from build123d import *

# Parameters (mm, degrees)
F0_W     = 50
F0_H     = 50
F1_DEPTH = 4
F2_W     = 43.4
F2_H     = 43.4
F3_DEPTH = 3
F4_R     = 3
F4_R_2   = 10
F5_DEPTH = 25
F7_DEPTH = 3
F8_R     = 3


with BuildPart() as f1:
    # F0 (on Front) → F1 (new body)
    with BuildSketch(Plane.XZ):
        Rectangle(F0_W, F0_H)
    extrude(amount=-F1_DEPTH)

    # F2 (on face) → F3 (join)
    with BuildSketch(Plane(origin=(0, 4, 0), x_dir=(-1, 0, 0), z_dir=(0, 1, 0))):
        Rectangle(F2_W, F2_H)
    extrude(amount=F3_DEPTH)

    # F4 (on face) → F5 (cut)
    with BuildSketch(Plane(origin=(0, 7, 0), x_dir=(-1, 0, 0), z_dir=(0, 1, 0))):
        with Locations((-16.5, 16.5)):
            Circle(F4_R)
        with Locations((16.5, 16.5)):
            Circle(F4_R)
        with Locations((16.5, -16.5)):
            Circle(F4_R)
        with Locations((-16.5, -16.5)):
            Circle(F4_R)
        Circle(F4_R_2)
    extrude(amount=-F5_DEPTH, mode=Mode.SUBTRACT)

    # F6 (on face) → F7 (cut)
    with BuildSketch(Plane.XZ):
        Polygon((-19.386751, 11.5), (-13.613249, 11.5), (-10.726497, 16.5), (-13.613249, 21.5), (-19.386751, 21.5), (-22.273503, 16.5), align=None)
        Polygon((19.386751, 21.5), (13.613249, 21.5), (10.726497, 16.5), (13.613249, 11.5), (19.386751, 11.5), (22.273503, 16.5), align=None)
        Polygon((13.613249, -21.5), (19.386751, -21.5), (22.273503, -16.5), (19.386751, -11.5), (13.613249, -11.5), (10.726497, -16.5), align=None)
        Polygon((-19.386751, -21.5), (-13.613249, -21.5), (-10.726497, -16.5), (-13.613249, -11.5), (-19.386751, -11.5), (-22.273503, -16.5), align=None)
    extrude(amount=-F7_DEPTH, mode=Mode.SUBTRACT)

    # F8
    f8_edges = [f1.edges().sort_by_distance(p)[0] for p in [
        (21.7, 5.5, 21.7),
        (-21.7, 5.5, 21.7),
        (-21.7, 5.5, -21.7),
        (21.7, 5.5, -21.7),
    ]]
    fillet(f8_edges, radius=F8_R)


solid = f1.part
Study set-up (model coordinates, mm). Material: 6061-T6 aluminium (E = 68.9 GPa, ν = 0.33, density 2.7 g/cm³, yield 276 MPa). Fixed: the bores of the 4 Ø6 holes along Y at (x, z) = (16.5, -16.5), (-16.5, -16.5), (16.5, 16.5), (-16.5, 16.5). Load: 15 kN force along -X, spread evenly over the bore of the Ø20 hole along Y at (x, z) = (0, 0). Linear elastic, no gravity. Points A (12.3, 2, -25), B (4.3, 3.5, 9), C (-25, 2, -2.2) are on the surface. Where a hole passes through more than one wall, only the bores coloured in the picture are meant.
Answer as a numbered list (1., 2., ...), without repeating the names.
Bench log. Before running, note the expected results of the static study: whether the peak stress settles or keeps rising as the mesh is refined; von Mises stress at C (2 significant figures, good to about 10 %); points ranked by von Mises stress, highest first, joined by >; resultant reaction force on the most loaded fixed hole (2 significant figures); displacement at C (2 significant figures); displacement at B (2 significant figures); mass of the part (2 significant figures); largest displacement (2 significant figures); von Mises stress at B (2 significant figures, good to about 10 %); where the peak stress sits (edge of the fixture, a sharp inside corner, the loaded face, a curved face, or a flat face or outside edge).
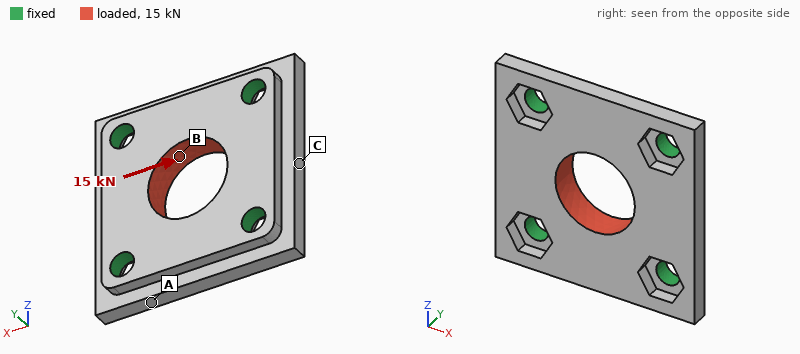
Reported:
1. keeps rising
2. 41 MPa
3. B > C > A
4. 3.9 kN
5. 15 µm
6. 12 µm
7. 32 g
8. 20 µm
9. 67 MPa
10. edge of the fixture
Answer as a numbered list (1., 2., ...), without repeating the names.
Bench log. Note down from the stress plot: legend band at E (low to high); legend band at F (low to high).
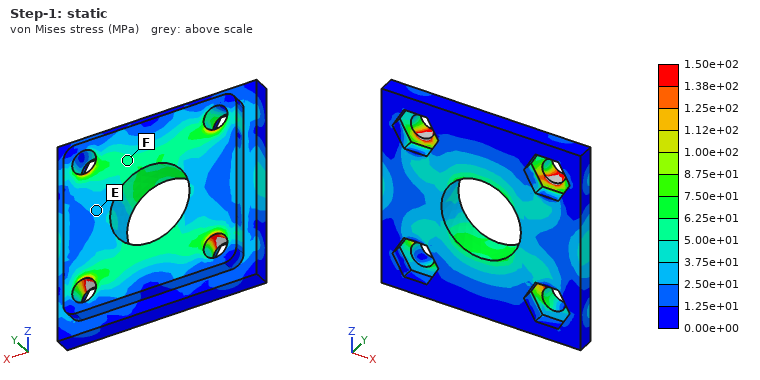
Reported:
1. 2.50e+01 to 3.75e+01 MPa
2. 5.00e+01 to 6.25e+01 MPa
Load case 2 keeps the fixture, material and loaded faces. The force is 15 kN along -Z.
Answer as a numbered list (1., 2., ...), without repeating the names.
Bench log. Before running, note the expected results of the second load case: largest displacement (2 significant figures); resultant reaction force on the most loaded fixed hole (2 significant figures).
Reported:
1. 20 µm
2. 3.9 kN
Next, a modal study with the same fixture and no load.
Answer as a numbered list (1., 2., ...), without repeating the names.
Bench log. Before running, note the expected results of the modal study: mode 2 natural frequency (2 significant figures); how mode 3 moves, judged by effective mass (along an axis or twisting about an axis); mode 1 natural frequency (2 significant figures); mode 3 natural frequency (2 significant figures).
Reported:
1. 23 kHz
2. twisting about X
3. 22 kHz
4. 25 kHz
